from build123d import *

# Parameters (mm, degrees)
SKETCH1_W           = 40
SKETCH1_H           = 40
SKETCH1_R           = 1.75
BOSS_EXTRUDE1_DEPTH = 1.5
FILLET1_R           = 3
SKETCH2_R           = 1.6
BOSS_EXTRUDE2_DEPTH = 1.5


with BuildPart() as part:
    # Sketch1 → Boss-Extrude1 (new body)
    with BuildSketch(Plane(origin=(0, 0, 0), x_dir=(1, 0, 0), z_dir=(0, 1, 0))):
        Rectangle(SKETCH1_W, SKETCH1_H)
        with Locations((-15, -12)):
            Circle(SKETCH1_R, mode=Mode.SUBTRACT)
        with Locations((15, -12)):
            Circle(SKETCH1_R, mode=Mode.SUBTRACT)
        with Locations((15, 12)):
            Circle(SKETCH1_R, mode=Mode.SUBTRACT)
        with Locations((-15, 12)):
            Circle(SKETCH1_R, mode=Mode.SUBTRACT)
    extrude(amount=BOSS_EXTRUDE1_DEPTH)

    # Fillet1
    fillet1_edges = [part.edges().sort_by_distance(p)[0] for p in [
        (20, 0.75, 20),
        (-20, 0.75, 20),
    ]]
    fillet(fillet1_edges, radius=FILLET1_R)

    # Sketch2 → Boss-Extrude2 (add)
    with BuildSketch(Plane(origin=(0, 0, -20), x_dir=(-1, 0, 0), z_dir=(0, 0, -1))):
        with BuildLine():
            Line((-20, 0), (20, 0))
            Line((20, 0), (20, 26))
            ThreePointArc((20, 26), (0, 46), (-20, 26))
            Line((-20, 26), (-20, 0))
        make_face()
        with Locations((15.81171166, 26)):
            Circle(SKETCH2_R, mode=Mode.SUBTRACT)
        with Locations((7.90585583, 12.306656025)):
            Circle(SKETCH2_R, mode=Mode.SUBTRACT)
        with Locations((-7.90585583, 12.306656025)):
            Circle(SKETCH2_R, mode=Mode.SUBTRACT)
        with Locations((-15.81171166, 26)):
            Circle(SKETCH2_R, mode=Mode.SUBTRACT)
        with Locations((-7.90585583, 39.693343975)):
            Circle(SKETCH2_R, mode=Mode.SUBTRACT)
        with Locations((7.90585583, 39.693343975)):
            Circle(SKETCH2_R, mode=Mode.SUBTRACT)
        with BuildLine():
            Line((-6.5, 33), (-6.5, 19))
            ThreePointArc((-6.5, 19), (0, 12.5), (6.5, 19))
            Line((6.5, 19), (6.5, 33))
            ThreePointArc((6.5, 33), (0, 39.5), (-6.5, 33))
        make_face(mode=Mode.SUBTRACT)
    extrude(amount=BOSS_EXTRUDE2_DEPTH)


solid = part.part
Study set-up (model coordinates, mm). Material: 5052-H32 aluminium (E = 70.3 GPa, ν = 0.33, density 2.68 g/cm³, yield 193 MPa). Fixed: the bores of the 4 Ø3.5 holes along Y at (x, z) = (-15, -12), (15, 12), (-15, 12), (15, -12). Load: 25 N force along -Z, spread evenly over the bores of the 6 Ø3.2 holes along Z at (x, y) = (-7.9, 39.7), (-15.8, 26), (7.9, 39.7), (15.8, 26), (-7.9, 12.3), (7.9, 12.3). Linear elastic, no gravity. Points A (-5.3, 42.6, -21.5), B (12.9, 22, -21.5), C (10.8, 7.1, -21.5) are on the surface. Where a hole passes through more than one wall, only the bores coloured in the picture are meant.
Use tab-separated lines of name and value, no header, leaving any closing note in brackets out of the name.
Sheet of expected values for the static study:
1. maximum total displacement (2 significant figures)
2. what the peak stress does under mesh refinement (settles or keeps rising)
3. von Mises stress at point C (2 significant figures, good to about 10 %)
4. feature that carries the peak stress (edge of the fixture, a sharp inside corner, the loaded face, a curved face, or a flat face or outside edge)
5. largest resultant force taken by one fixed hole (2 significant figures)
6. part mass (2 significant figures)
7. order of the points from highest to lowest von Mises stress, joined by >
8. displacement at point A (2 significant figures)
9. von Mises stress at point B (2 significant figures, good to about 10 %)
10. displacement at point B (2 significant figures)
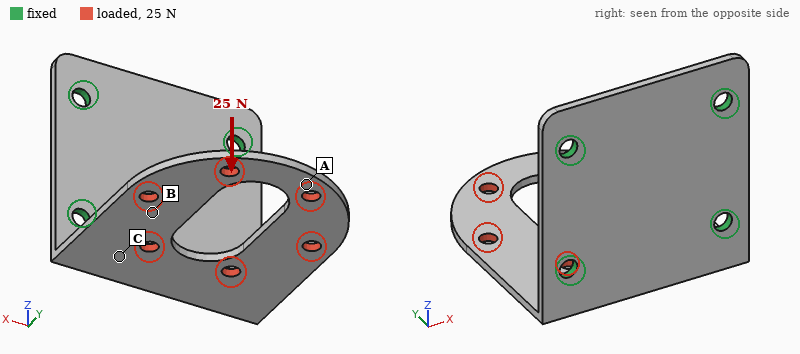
maximum total displacement	0.75 mm
what the peak stress does under mesh refinement	keeps rising
von Mises stress at point C	29 MPa
feature that carries the peak stress	edge of the fixture
largest resultant force taken by one fixed hole	8.8 N
part mass	12 g
order of the points from highest to lowest von Mises stress, joined by >	C > B > A
displacement at point A	0.68 mm
von Mises stress at point B	19 MPa
displacement at point B	0.27 mm
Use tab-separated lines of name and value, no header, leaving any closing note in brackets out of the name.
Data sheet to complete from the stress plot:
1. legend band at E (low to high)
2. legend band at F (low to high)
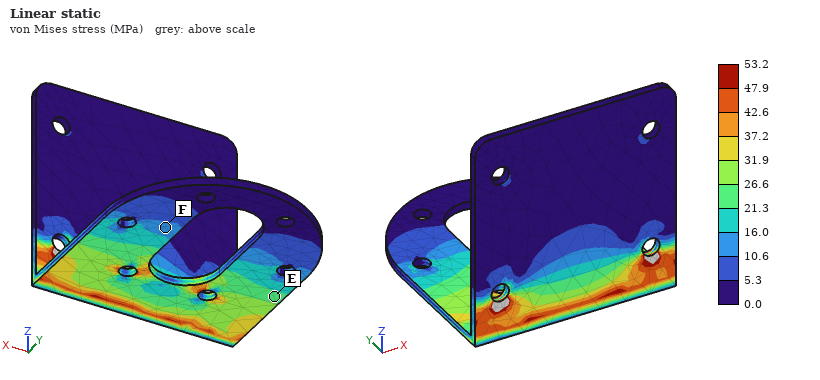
legend band at E	21.3 to 26.6 MPa
legend band at F	10.6 to 16.0 MPa
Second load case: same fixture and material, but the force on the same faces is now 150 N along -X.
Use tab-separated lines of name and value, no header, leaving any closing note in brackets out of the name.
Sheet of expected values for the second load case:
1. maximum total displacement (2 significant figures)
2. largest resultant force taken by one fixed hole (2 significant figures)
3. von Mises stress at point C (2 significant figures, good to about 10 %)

maximum total displacement	0.17 mm
largest resultant force taken by one fixed hole	150 N
von Mises stress at point C	19 MPa
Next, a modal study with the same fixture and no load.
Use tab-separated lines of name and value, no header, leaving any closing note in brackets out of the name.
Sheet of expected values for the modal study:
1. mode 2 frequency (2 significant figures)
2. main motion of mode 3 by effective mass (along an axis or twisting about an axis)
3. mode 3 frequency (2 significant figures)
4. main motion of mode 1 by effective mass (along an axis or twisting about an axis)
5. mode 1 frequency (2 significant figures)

mode 2 frequency	1600 Hz
main motion of mode 3 by effective mass	along X
mode 3 frequency	3000 Hz
main motion of mode 1 by effective mass	along Z
mode 1 frequency	610 Hz
